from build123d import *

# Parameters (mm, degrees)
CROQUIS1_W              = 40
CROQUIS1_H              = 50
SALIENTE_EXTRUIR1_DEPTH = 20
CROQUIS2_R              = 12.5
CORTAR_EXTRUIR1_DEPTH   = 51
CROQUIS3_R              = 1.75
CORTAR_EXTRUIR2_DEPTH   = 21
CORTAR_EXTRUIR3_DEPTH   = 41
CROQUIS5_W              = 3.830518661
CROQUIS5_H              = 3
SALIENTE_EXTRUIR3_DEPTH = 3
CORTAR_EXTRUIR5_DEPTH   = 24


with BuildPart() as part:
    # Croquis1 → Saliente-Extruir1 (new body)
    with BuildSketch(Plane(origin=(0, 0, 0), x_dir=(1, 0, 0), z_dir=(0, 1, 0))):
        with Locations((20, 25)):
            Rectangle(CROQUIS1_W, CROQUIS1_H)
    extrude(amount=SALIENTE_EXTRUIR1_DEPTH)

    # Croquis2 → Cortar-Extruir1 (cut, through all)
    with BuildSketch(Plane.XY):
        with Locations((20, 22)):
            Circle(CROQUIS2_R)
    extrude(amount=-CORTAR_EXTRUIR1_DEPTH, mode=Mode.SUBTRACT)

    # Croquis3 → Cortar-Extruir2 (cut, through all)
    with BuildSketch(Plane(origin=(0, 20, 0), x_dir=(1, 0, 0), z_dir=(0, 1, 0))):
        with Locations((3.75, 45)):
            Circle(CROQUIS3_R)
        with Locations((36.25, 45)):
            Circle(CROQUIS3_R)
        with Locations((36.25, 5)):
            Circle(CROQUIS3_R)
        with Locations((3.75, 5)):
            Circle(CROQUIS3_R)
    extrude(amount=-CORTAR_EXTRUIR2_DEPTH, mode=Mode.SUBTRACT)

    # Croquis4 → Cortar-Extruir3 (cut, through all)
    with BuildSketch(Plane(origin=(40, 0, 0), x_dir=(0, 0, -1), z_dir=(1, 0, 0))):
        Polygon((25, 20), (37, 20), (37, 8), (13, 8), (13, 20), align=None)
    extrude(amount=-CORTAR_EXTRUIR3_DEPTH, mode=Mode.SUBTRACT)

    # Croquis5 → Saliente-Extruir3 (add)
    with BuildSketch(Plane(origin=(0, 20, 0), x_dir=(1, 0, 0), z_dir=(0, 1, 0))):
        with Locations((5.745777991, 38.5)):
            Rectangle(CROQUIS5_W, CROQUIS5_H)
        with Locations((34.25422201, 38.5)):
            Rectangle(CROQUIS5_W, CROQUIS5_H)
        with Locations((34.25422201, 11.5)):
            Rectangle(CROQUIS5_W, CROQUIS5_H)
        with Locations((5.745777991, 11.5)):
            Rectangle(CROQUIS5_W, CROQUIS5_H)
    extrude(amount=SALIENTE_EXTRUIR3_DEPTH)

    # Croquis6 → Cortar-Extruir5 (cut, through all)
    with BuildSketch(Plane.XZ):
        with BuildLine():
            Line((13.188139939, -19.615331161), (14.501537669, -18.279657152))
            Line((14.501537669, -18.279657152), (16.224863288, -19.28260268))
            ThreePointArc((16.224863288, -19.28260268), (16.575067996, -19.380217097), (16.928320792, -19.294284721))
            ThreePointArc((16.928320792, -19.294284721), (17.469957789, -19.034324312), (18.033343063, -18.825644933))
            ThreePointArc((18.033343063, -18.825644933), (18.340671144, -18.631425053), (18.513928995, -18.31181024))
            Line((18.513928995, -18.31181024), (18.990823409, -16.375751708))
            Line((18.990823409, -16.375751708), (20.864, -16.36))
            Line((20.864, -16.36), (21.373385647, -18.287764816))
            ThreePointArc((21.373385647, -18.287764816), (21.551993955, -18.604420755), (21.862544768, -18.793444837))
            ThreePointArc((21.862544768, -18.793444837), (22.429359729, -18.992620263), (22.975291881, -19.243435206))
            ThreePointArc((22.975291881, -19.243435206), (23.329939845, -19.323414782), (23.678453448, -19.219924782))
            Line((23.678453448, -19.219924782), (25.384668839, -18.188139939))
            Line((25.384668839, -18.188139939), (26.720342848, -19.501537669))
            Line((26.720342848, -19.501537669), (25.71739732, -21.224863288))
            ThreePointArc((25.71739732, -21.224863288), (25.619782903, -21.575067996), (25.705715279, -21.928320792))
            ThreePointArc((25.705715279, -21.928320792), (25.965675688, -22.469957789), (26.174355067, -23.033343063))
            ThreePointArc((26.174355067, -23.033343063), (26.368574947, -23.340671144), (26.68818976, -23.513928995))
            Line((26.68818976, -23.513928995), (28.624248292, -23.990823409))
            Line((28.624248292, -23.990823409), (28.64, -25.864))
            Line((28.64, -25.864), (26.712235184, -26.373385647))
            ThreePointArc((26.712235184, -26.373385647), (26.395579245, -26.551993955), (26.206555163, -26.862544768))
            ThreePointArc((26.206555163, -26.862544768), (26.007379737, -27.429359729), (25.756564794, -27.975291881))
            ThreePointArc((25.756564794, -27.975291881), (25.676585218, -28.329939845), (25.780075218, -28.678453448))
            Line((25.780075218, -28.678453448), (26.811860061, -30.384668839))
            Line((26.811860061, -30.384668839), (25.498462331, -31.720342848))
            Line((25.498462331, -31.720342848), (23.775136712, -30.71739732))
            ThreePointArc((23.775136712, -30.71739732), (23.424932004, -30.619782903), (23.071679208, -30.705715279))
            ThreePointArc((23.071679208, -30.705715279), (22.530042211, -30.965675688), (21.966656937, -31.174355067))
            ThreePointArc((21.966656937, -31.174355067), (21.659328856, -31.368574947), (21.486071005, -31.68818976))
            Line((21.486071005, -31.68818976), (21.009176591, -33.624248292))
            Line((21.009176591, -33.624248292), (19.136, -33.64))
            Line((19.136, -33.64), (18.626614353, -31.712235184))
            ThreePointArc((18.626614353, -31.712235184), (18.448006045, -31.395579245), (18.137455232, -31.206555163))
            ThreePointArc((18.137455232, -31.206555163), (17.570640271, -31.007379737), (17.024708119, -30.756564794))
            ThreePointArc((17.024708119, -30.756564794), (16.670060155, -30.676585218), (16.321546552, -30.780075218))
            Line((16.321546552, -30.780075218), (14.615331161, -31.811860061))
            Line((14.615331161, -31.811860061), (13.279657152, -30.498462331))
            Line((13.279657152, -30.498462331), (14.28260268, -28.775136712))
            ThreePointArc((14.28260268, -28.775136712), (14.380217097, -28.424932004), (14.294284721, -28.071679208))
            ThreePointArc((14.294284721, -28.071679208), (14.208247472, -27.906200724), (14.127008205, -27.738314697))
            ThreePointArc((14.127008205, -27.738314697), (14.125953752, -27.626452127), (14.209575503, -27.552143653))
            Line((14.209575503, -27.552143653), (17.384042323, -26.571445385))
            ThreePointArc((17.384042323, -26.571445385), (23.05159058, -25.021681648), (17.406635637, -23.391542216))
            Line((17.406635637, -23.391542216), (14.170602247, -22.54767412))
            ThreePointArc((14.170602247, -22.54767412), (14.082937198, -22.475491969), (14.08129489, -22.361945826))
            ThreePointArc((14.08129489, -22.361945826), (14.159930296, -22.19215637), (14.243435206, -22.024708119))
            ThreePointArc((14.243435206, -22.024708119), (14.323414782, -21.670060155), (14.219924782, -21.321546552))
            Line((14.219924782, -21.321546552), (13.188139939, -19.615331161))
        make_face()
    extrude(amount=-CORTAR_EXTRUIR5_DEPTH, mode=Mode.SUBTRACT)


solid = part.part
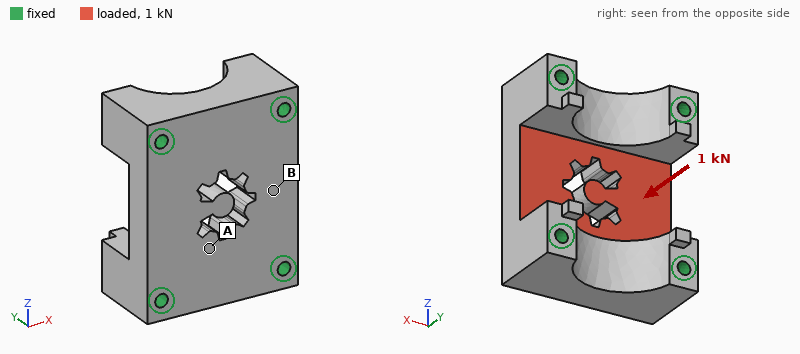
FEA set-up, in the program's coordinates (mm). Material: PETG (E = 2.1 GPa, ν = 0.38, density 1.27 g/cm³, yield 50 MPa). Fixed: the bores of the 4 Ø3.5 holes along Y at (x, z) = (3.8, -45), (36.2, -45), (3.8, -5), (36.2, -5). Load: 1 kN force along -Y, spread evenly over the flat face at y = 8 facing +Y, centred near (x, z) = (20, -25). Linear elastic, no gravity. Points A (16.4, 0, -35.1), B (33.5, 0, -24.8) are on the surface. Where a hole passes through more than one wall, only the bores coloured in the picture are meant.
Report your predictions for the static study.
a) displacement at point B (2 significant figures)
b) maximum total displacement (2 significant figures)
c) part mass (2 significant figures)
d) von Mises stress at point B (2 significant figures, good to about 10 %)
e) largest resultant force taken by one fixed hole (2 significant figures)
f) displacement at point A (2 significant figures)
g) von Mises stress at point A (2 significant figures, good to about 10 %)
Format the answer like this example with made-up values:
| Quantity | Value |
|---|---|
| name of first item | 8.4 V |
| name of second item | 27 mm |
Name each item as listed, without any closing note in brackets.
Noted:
| Quantity | Value |
|---|---|
| displacement at point B | 0.067 mm |
| maximum total displacement | 0.20 mm |
| part mass | 28 g |
| von Mises stress at point B | 5.7 MPa |
| largest resultant force taken by one fixed hole | 270 N |
| displacement at point A | 0.055 mm |
| von Mises stress at point A | 2.0 MPa |
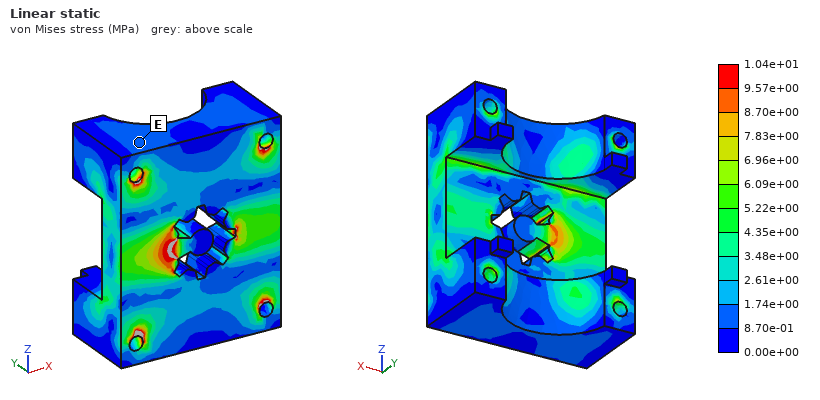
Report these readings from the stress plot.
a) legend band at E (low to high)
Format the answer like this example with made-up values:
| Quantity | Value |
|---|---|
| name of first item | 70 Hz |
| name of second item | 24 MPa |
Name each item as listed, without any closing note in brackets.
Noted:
| Quantity | Value |
|---|---|
| legend band at E | 8.70e-01 to 1.74e+00 MPa |
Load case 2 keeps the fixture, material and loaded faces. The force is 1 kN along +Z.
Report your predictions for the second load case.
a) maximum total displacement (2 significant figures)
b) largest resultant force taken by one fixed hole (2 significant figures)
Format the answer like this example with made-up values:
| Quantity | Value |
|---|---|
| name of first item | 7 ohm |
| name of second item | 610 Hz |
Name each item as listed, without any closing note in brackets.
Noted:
| Quantity | Value |
|---|---|
| maximum total displacement | 0.14 mm |
| largest resultant force taken by one fixed hole | 280 N |
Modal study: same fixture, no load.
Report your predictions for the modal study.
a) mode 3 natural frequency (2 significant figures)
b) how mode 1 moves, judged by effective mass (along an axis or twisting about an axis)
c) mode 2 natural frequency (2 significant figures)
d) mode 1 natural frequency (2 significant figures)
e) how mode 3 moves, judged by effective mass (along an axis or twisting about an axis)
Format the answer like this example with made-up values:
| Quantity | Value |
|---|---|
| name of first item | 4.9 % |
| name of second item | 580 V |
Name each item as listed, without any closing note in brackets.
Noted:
| Quantity | Value |
|---|---|
| mode 3 natural frequency | 7400 Hz |
| how mode 1 moves, judged by effective mass | along Y |
| mode 2 natural frequency | 7000 Hz |
| mode 1 natural frequency | 5400 Hz |
| how mode 3 moves, judged by effective mass | along Y |
